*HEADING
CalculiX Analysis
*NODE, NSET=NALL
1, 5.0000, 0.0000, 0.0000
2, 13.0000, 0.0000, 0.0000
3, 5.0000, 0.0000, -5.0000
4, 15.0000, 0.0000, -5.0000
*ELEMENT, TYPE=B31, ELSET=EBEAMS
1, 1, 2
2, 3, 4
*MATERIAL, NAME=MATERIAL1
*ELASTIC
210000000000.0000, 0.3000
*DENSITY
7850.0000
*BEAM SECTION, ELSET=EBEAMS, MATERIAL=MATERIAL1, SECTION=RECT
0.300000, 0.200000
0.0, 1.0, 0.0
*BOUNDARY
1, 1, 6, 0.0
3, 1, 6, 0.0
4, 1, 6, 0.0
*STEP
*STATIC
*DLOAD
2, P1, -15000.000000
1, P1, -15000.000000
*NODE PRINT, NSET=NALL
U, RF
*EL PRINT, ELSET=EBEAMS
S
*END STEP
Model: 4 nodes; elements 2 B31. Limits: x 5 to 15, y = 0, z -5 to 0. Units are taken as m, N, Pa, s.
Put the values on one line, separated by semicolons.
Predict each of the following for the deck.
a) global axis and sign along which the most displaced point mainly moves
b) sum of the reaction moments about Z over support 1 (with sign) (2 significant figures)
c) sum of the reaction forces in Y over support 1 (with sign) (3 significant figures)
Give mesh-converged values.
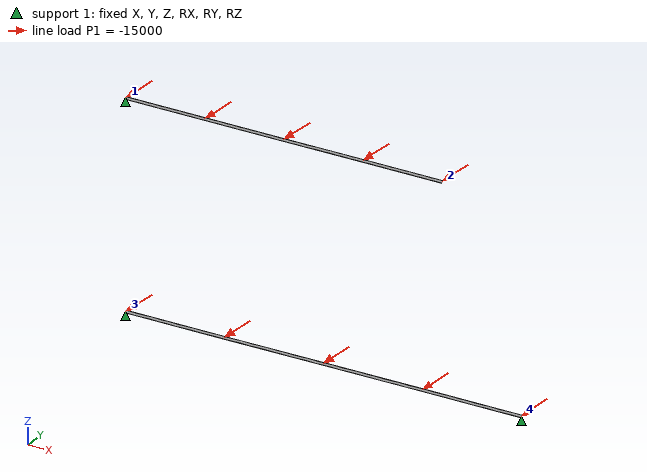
-Y; 4.8e+05 N·m; 2.70e+05 N
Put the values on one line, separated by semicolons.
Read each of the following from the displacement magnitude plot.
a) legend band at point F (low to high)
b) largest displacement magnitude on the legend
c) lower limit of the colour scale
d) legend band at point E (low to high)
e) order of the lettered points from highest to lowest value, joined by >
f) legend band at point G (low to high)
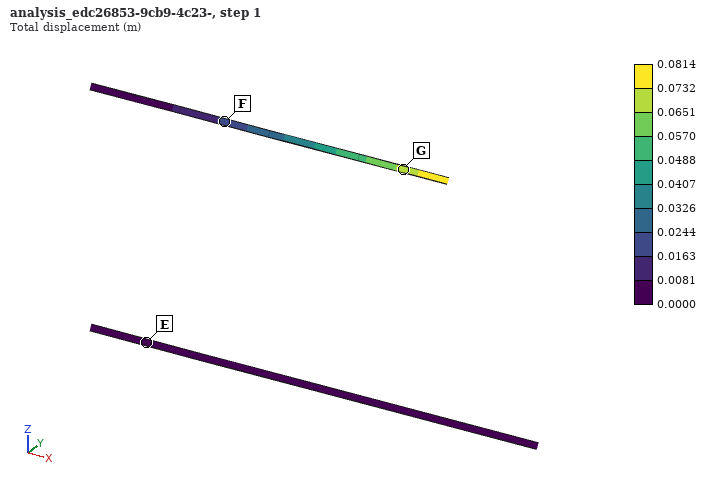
0.0163 to 0.0244 m; 0.0814 m; 0.0000 m; 0.0000 to 0.0081 m; G > F > E; 0.0651 to 0.0732 m
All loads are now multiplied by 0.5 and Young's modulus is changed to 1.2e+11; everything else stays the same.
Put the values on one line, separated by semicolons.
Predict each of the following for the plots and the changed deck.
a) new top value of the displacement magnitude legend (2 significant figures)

0.071 m
